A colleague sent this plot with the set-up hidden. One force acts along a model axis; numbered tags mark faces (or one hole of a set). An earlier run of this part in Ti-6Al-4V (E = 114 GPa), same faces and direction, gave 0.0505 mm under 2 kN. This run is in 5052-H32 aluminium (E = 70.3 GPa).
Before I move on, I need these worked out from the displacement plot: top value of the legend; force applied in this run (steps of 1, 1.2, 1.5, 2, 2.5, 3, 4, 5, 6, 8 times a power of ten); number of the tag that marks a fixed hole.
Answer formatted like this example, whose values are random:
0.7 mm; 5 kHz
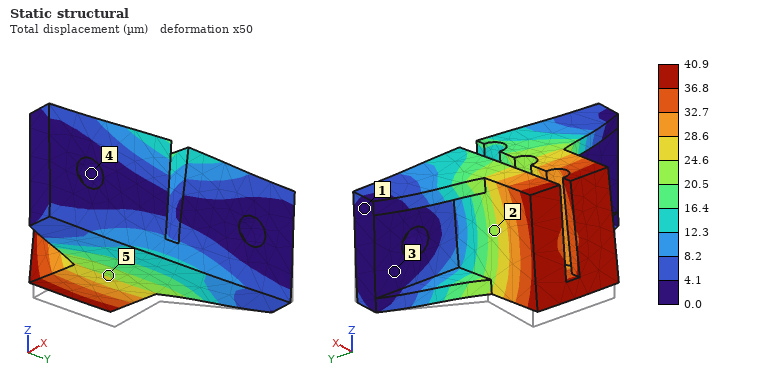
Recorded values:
40.9 µm; 1 kN; 4
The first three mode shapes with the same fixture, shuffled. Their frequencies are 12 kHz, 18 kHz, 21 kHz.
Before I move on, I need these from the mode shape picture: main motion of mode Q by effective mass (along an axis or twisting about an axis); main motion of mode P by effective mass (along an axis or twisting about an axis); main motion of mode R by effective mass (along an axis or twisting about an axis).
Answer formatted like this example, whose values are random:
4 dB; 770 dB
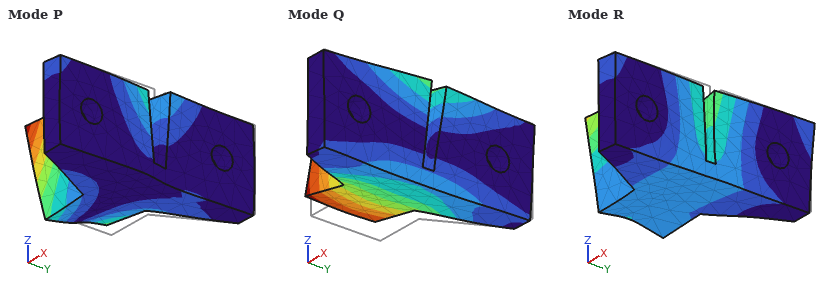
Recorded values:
along Z; along Y; along X
